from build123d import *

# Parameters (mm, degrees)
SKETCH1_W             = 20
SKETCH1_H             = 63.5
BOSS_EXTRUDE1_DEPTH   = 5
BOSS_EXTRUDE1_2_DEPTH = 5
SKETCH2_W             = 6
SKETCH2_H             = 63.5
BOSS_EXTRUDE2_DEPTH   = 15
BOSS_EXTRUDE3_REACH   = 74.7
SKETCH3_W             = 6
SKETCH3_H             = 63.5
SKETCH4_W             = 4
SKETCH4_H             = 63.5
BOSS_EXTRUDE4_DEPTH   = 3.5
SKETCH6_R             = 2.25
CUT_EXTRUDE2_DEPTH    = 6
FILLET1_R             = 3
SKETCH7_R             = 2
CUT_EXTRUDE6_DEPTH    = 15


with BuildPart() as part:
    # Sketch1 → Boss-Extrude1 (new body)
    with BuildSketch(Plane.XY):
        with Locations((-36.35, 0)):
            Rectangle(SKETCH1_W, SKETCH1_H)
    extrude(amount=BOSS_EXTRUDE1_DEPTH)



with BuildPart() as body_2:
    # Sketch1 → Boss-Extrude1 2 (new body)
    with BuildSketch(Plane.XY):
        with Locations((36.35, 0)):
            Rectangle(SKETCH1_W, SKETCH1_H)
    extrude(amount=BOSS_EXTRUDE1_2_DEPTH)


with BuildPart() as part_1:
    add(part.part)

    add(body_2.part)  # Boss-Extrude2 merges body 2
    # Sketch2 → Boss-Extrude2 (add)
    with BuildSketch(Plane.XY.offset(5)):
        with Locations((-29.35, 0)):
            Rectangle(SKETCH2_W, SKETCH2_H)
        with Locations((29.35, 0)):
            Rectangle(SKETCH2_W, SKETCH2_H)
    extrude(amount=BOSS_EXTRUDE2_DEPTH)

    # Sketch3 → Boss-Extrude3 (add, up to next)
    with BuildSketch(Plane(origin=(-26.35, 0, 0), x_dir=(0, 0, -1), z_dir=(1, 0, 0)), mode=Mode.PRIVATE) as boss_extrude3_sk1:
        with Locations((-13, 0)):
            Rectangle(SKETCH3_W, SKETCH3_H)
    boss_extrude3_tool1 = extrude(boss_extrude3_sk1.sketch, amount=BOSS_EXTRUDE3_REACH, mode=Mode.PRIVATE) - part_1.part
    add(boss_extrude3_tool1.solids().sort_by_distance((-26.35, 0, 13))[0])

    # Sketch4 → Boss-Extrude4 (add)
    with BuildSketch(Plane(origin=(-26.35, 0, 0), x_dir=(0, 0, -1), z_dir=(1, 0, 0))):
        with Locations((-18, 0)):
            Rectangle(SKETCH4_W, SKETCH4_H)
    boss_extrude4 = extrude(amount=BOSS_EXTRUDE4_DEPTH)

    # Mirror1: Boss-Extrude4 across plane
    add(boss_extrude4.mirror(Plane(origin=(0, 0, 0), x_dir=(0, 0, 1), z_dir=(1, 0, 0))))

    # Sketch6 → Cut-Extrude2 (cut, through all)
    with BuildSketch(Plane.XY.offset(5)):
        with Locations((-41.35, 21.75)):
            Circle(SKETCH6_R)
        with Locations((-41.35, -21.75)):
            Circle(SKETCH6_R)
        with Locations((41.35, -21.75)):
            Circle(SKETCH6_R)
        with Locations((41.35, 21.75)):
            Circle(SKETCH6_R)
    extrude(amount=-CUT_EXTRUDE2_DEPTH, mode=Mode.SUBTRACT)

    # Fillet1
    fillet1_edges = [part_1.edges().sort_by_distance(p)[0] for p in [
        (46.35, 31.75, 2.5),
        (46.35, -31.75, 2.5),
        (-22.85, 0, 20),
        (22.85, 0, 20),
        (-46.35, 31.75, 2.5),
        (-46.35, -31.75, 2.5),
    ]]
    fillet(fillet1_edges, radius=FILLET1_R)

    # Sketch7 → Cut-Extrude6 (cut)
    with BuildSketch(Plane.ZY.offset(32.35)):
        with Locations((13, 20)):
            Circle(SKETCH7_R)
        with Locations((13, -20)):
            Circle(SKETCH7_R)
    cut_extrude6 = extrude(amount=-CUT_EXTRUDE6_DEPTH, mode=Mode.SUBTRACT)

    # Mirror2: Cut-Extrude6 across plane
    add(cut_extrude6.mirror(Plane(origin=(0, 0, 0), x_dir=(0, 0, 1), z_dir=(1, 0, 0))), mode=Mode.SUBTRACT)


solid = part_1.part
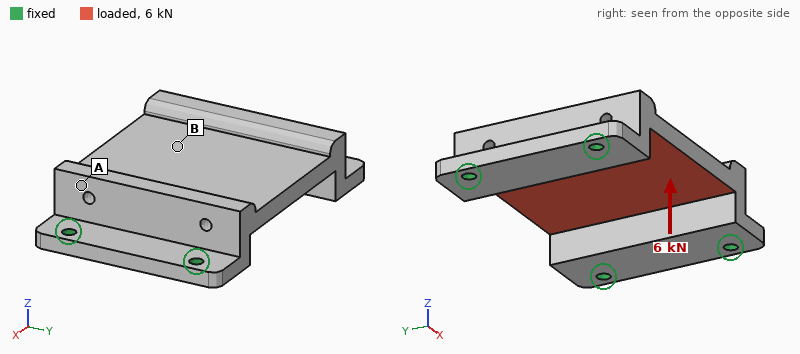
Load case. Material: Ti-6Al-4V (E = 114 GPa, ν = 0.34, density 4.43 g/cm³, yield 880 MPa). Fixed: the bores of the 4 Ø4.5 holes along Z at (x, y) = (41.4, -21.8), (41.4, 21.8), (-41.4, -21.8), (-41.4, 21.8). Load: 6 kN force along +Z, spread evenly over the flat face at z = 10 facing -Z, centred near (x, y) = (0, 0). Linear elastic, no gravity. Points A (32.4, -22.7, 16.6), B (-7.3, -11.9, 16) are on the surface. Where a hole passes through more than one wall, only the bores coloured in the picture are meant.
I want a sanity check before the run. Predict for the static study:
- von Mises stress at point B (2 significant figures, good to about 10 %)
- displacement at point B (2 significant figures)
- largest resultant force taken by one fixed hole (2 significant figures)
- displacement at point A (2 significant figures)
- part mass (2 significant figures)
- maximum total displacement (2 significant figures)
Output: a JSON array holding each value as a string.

["48 MPa", "46 µm", "2.8 kN", "13 µm", "200 g", "53 µm"]
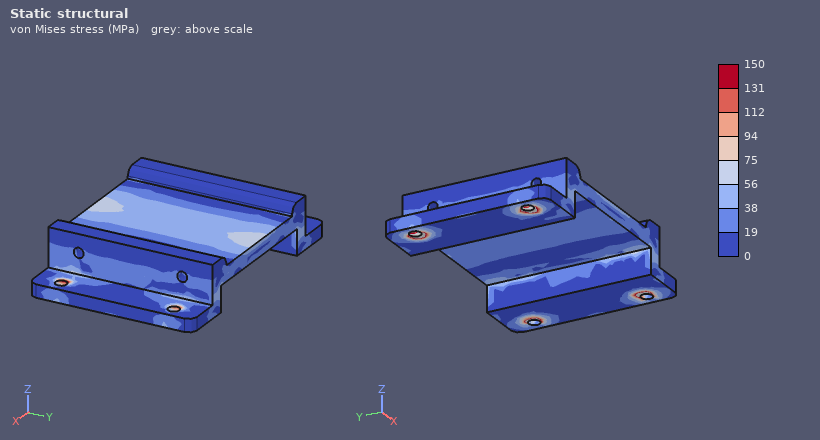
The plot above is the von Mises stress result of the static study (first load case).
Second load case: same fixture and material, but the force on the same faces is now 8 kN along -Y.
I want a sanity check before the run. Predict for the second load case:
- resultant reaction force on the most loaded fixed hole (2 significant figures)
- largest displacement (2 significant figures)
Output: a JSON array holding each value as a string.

["2.4 kN", "17 µm"]
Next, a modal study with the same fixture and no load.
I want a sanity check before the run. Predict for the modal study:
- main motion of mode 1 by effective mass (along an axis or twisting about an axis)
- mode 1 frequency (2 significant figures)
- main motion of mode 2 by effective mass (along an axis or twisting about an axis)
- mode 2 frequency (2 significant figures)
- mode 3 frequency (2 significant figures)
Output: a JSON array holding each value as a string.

["along Z", "6000 Hz", "along X", "6700 Hz", "7100 Hz"]
